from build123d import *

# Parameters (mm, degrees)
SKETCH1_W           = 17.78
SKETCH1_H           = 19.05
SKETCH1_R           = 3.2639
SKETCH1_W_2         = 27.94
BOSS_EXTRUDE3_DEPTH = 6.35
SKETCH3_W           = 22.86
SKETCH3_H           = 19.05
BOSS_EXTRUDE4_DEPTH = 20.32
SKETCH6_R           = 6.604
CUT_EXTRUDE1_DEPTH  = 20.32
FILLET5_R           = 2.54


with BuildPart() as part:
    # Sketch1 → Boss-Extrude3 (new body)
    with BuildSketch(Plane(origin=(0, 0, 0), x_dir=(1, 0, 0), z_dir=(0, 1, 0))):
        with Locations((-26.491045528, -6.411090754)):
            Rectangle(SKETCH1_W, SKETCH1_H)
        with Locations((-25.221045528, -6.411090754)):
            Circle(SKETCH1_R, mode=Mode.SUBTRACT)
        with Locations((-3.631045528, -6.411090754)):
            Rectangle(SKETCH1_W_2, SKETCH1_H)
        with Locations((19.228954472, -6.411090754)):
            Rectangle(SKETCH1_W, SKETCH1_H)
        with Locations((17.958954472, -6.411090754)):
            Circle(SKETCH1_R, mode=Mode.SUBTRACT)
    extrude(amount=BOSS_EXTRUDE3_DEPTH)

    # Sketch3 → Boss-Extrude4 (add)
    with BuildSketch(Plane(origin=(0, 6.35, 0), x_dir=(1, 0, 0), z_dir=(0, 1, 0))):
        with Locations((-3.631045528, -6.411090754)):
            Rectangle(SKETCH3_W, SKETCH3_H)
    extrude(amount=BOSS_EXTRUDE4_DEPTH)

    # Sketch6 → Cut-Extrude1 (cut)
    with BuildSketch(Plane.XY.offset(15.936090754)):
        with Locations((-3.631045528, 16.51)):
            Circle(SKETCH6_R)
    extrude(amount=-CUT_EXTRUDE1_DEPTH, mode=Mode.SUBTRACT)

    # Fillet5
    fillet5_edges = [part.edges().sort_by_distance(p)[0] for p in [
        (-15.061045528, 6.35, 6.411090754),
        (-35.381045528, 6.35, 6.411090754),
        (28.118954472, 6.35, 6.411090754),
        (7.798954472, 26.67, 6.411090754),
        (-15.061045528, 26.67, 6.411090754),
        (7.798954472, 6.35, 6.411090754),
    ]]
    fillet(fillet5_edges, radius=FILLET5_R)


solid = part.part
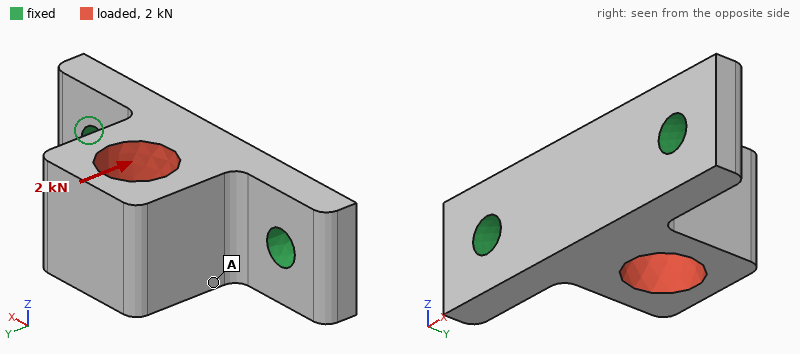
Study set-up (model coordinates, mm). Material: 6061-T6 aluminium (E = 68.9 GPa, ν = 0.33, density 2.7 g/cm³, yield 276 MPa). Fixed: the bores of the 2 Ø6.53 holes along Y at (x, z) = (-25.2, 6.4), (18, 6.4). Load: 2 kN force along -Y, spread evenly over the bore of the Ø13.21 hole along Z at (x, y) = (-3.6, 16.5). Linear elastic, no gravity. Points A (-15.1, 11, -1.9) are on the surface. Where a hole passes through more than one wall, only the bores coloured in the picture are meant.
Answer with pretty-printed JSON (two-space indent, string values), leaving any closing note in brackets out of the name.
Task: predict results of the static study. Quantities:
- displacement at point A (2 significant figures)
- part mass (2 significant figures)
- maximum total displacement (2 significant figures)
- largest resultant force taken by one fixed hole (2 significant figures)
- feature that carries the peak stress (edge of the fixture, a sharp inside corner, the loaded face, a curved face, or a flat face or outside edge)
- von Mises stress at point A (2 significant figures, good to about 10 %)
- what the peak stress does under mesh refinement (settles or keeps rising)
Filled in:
{
  "displacement at point A": "8.7 µm",
  "part mass": "36 g",
  "maximum total displacement": "10 µm",
  "largest resultant force taken by one fixed hole": "1.1 kN",
  "feature that carries the peak stress": "edge of the fixture",
  "von Mises stress at point A": "12 MPa",
  "what the peak stress does under mesh refinement": "keeps rising"
}
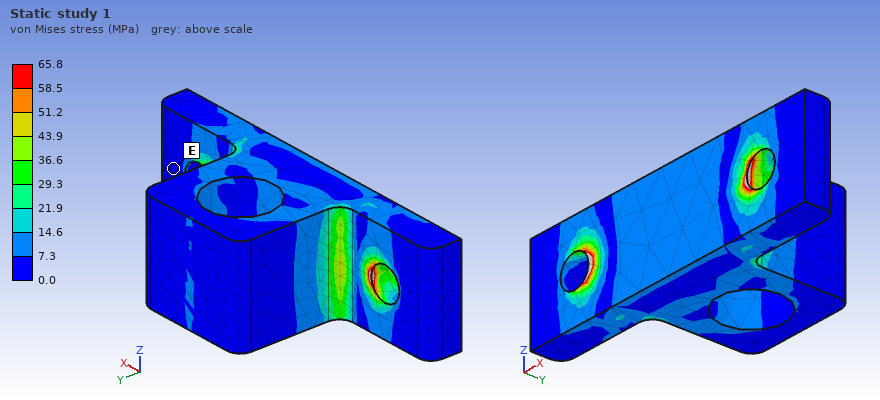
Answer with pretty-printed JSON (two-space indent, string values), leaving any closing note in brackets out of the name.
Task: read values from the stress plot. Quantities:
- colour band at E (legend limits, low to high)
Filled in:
{
  "colour band at E": "0.0 to 7.3 MPa"
}
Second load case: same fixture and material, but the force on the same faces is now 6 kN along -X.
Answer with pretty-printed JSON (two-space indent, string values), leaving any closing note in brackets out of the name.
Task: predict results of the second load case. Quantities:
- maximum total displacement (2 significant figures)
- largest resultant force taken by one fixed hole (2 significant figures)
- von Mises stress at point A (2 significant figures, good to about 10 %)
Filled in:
{
  "maximum total displacement": "64 µm",
  "largest resultant force taken by one fixed hole": "3.9 kN",
  "von Mises stress at point A": "65 MPa"
}
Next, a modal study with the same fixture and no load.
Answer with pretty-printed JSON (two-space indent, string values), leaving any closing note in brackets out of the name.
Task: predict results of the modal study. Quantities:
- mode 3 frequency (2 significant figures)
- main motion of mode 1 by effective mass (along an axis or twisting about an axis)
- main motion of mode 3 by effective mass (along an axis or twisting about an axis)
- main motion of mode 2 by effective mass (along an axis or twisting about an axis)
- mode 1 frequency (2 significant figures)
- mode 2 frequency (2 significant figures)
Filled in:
{
  "mode 3 frequency": "15 kHz",
  "main motion of mode 1 by effective mass": "along Z",
  "main motion of mode 3 by effective mass": "along Y",
  "main motion of mode 2 by effective mass": "along X",
  "mode 1 frequency": "6600 Hz",
  "mode 2 frequency": "13 kHz"
}
